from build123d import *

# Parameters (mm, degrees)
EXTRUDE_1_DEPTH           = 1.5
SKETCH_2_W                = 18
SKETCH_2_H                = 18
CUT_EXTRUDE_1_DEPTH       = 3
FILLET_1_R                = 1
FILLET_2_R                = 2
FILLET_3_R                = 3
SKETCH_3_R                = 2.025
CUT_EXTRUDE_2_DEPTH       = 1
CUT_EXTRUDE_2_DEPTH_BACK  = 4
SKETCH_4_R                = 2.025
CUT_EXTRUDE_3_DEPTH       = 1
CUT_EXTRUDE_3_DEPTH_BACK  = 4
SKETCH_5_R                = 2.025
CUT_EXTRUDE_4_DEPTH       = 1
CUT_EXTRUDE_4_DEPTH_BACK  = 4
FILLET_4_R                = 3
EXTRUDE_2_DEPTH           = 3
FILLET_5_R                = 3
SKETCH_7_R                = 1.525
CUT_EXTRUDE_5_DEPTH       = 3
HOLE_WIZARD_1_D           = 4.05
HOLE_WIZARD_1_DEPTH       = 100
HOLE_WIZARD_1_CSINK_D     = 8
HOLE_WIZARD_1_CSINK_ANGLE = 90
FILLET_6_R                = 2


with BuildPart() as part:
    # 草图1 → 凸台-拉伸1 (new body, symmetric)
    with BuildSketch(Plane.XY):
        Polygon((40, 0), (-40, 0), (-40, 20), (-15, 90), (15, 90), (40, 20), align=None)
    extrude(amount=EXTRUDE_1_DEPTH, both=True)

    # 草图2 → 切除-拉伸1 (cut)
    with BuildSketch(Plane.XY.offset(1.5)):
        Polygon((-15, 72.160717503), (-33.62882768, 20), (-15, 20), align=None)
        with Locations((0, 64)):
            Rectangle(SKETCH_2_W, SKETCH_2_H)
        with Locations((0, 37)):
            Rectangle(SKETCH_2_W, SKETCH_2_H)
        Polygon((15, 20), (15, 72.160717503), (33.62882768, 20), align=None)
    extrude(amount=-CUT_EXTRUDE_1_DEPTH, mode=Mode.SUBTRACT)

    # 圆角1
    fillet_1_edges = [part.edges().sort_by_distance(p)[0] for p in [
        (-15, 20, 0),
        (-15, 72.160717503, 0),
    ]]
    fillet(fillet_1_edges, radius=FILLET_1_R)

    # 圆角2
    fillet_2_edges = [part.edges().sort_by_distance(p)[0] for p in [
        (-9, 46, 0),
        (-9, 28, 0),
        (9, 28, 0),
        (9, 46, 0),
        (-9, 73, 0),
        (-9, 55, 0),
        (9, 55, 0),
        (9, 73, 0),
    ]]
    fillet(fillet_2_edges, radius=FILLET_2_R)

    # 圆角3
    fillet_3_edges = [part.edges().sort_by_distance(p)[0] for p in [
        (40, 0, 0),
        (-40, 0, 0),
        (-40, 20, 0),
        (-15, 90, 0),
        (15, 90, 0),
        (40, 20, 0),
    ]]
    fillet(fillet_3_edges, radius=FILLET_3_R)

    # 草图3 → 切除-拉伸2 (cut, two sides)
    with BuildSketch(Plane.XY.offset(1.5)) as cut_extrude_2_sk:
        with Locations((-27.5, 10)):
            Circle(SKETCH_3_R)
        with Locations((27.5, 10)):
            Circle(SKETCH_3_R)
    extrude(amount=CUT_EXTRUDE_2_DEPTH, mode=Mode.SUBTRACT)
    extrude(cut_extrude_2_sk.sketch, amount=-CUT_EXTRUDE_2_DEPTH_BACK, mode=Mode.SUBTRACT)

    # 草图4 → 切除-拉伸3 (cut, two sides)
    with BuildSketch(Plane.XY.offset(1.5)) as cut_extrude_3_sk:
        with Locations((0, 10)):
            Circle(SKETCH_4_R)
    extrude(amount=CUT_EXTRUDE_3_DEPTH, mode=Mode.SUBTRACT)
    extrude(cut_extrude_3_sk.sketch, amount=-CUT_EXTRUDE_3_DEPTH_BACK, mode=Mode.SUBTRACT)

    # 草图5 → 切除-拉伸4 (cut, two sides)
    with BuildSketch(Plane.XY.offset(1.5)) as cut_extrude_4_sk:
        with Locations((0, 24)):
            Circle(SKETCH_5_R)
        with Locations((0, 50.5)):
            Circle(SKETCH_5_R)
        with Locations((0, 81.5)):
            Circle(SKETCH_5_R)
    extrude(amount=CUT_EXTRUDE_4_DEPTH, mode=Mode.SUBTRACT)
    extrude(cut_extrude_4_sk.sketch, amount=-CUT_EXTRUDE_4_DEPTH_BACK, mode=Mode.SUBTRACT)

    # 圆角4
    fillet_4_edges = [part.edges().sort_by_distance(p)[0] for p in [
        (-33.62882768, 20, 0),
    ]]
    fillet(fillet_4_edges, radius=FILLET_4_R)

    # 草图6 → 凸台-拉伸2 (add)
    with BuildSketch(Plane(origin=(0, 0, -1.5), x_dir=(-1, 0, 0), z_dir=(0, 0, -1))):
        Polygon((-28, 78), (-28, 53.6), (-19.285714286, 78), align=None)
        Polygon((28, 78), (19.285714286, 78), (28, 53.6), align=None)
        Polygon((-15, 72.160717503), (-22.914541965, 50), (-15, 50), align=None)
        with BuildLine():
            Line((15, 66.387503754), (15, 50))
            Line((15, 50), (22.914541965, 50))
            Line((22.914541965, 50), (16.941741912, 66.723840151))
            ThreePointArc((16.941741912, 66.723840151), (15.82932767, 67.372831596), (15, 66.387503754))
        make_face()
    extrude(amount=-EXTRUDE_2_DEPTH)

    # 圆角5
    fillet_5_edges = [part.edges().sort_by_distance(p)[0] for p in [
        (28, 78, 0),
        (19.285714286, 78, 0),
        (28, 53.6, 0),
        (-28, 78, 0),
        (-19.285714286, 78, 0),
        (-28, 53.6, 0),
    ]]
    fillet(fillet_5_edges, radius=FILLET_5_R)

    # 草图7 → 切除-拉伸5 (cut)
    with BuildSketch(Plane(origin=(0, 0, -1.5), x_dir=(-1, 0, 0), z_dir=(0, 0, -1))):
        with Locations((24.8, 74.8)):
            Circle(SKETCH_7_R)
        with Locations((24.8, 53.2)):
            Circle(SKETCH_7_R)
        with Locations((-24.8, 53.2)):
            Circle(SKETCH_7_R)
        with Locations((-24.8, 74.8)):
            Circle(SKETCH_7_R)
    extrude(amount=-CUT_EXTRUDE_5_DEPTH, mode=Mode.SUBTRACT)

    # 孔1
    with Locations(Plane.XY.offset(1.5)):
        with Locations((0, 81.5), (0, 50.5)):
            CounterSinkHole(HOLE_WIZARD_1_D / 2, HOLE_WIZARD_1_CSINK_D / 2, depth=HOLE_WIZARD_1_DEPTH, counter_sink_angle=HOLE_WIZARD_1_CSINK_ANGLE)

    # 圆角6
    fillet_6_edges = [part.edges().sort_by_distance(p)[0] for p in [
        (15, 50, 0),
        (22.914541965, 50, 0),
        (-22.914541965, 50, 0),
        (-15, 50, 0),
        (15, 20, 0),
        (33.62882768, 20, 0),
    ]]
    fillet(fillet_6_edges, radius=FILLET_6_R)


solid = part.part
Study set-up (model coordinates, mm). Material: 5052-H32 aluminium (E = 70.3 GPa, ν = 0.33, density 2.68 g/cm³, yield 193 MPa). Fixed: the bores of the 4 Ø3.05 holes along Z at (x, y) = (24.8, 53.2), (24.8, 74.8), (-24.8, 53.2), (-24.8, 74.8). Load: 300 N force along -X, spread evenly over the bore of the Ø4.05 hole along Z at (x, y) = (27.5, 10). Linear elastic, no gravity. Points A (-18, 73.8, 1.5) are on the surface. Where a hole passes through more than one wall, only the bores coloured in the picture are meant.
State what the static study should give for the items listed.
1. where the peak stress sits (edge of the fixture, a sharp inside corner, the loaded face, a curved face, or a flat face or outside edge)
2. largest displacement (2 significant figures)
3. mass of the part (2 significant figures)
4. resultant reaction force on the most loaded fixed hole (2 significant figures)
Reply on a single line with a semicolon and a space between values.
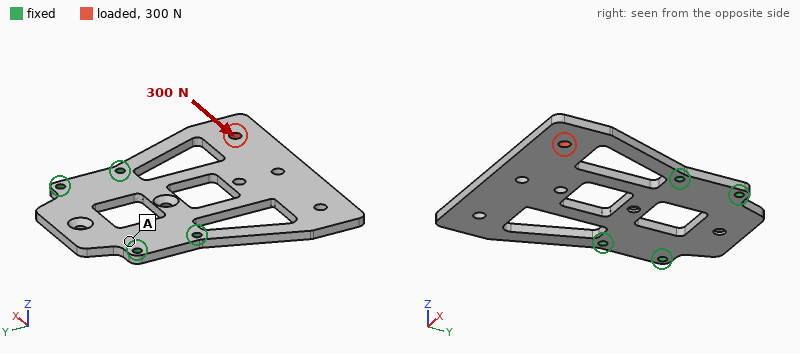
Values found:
a curved face; 66 µm; 33 g; 220 N
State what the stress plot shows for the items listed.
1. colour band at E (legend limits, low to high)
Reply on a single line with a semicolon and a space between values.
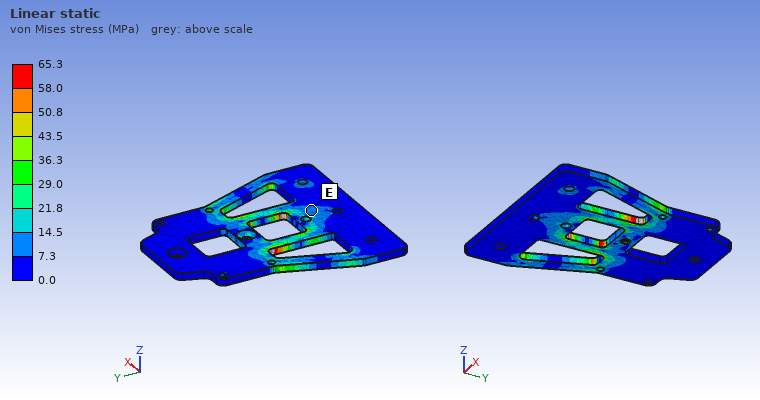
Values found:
7.3 to 14.5 MPa
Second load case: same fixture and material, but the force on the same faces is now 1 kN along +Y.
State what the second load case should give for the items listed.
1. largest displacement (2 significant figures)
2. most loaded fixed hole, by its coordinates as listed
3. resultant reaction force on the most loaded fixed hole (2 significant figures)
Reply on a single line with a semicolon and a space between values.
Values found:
61 µm; (24.8, 53.2); 870 N
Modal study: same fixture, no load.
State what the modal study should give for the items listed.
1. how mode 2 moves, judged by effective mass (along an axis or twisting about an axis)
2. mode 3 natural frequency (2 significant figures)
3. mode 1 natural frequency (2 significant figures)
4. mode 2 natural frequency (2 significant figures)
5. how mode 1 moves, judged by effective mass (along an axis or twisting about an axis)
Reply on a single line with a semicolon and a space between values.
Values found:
twisting about Y; 2700 Hz; 500 Hz; 1100 Hz; along Z
